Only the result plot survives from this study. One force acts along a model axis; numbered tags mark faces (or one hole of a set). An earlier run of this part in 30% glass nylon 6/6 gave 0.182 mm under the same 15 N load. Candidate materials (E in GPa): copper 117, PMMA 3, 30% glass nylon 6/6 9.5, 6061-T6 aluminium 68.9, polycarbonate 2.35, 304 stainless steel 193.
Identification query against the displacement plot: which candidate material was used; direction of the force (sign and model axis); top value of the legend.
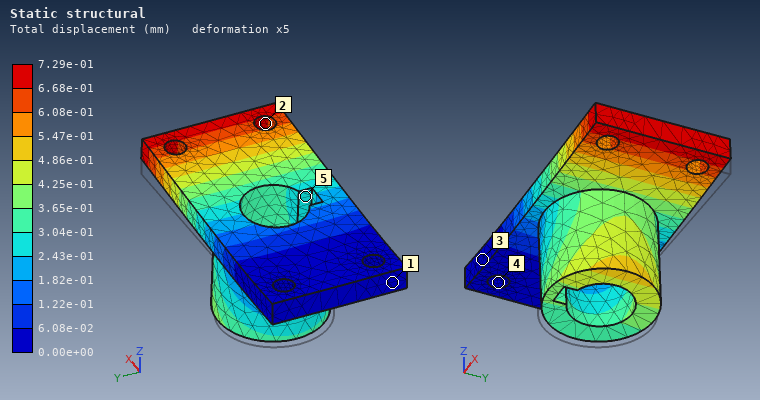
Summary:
polycarbonate
+Z
7.29e-01 mm
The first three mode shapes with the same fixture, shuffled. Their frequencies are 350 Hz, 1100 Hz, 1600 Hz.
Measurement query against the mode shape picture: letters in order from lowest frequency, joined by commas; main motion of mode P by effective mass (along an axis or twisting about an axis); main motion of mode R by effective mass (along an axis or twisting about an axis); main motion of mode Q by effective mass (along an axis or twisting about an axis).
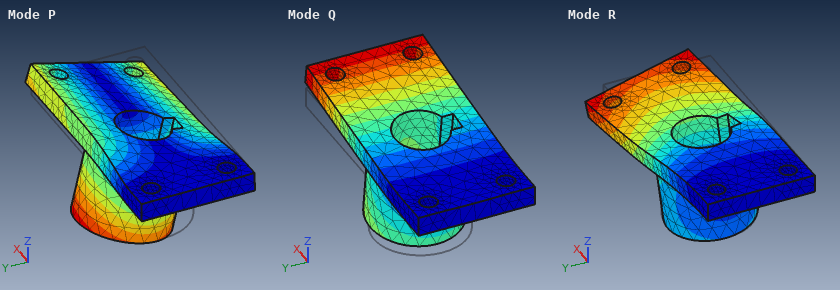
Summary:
Q, P, R
along Y
along Y
along Z
